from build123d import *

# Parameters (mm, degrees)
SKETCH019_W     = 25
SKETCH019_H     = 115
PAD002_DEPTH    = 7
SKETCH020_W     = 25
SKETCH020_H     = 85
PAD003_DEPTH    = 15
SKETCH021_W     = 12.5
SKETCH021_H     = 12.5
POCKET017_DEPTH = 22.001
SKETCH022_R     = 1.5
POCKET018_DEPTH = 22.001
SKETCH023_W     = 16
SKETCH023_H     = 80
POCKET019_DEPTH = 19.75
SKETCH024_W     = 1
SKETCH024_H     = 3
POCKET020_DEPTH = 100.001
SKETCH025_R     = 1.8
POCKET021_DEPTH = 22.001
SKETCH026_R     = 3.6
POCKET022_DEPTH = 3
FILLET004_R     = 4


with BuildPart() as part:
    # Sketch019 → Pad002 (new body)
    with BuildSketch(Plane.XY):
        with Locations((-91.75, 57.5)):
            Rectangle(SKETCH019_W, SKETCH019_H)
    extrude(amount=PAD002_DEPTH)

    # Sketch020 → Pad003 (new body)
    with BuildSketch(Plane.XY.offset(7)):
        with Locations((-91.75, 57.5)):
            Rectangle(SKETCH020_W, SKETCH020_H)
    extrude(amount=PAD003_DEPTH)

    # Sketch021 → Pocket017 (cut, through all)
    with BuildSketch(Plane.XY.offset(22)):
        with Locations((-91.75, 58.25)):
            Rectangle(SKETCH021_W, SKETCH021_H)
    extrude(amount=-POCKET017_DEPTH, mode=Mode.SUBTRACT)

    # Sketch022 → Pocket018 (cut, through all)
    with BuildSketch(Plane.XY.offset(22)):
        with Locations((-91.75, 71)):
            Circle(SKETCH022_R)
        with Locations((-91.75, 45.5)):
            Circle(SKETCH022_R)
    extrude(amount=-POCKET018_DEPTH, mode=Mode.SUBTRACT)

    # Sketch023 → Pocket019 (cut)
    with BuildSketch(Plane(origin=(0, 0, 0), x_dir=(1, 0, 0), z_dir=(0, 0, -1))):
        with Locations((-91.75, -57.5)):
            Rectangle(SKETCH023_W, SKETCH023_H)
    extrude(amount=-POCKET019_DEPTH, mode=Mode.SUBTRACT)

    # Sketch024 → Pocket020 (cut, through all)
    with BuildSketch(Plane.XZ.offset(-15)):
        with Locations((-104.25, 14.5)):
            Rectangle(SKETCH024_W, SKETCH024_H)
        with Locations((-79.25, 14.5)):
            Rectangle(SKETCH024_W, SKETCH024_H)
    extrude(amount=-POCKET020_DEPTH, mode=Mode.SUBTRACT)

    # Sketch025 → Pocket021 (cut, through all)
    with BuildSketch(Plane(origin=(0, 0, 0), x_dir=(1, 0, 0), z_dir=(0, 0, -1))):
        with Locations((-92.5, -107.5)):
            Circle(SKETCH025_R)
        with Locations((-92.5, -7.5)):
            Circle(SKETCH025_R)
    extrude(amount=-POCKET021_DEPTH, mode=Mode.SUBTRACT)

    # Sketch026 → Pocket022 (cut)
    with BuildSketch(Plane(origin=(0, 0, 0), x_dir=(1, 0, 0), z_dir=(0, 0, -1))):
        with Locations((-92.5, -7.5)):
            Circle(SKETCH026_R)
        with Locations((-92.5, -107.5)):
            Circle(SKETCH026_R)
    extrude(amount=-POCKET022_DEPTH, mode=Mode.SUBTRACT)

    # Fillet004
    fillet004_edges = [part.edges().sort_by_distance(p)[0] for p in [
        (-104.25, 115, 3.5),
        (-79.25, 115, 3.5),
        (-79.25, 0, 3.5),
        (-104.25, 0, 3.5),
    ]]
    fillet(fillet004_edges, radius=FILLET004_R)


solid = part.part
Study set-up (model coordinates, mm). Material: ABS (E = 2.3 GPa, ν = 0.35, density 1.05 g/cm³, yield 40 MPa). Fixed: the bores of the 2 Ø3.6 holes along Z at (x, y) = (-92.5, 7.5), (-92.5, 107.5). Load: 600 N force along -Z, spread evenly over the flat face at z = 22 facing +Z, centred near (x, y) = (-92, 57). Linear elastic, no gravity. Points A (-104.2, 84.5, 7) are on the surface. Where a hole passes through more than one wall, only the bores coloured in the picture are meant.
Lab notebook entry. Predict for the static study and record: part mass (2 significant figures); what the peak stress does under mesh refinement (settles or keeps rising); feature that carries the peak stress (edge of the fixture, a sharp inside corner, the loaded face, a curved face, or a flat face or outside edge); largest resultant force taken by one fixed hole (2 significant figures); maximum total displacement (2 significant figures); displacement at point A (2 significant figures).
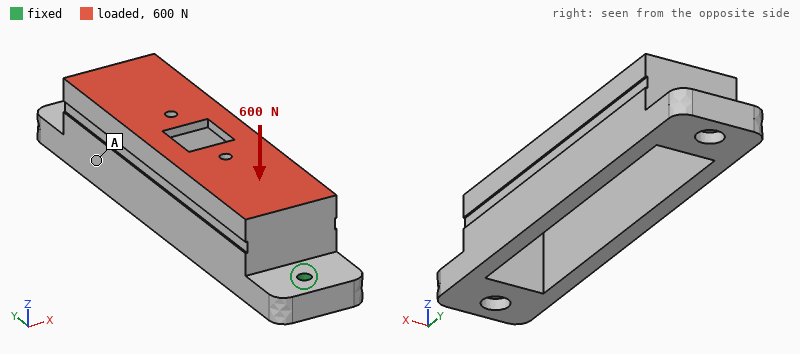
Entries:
27 g
keeps rising
edge of the fixture
360 N
0.48 mm
0.25 mm
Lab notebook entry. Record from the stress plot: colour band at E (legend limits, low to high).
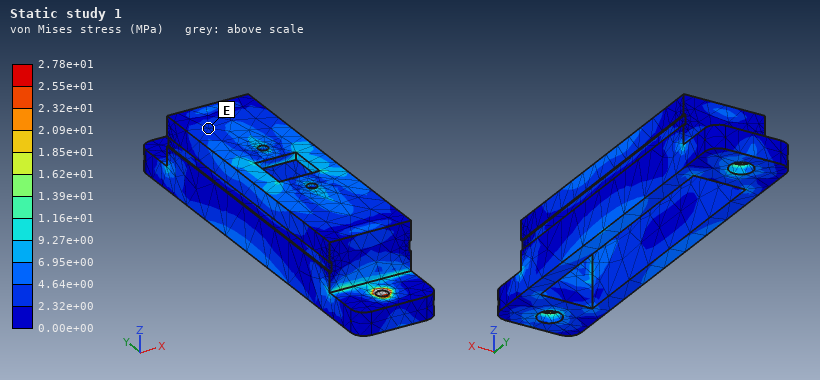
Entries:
2.32e+00 to 4.64e+00 MPa
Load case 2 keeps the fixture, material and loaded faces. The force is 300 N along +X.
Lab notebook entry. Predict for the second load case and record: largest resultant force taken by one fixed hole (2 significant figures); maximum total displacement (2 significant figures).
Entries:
150 N
0.83 mm
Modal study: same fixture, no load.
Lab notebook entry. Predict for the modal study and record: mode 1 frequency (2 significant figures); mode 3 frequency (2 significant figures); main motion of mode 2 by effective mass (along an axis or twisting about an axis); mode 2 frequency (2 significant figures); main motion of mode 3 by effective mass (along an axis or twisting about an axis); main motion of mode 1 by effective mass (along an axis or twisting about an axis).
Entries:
920 Hz
1500 Hz
along X
1300 Hz
along Z
along X
